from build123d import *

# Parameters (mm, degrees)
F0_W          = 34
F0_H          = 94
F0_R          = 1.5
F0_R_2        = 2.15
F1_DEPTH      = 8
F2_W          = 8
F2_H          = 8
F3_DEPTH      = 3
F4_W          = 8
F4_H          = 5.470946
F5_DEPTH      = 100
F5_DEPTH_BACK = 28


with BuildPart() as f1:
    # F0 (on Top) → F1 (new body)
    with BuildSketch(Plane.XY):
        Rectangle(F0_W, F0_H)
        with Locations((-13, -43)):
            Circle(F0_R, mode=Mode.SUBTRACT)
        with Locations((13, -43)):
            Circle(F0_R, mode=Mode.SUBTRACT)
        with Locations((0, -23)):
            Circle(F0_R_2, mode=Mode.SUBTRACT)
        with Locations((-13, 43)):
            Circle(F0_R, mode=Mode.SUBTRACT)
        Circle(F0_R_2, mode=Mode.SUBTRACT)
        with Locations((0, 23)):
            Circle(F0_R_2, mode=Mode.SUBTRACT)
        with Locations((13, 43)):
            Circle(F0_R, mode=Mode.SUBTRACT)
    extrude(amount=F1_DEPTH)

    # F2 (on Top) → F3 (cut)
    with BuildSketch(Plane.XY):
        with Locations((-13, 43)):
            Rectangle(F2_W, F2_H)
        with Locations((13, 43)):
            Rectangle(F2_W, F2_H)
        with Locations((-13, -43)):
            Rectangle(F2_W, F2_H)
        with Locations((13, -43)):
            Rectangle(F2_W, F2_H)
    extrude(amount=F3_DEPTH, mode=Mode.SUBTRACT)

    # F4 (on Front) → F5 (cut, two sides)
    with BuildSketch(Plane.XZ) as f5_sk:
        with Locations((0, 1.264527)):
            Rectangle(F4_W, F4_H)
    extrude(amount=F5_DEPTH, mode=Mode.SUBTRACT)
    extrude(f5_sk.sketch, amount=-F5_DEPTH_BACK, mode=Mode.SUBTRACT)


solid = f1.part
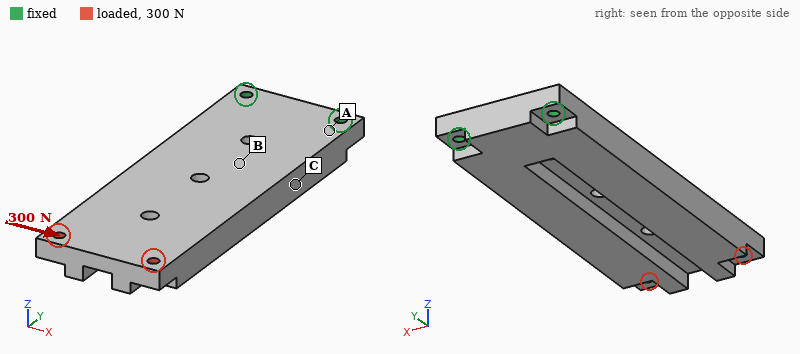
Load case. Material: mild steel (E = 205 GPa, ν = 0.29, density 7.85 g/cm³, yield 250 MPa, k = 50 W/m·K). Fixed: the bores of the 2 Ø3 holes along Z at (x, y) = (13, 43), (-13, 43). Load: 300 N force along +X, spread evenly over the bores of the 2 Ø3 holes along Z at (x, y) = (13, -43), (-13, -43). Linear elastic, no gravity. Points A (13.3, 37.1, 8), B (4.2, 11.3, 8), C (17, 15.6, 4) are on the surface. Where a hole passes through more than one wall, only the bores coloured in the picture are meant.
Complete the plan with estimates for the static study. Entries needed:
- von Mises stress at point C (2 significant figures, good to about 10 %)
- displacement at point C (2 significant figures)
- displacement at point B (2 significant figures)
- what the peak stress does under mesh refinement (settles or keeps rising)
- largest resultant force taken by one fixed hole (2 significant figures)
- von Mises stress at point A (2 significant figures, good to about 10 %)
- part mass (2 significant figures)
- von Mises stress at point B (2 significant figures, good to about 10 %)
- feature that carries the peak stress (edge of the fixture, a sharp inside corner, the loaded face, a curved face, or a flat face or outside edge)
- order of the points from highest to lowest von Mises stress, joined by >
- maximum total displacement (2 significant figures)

12 MPa
4.1 µm
4.0 µm
keeps rising
980 N
19 MPa
170 g
5.5 MPa
edge of the fixture
A > C > B
18 µm
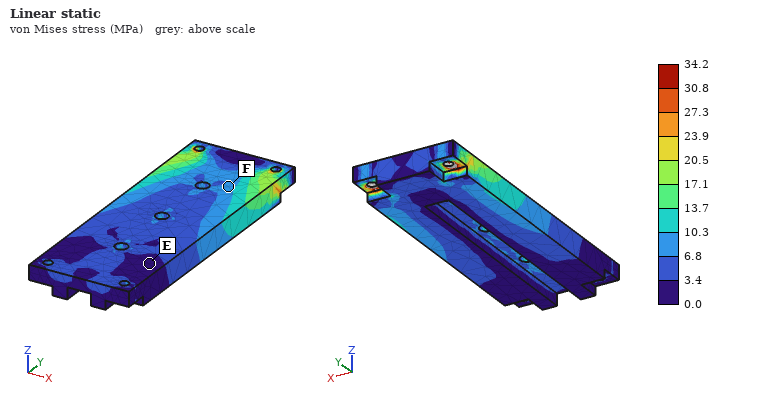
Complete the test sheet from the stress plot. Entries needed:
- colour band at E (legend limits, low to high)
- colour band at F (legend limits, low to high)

0.0 to 3.4 MPa
6.8 to 10.3 MPa
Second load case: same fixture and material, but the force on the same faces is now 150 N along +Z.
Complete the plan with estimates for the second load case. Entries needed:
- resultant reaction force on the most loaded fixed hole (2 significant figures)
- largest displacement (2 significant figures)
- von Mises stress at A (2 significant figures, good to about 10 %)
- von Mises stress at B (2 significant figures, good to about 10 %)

99 N
0.21 mm
61 MPa
23 MPa
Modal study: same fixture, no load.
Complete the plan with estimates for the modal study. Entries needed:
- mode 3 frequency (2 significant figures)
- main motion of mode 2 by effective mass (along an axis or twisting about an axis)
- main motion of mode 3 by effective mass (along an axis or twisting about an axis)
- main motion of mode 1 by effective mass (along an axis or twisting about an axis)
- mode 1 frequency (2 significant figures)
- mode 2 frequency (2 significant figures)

3400 Hz
along X
twisting about Y
along Z
640 Hz
3000 Hz
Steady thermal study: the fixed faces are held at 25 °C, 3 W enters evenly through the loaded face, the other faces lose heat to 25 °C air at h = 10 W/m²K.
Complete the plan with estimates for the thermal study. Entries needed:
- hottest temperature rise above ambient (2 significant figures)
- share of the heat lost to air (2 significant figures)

21 K
28 %
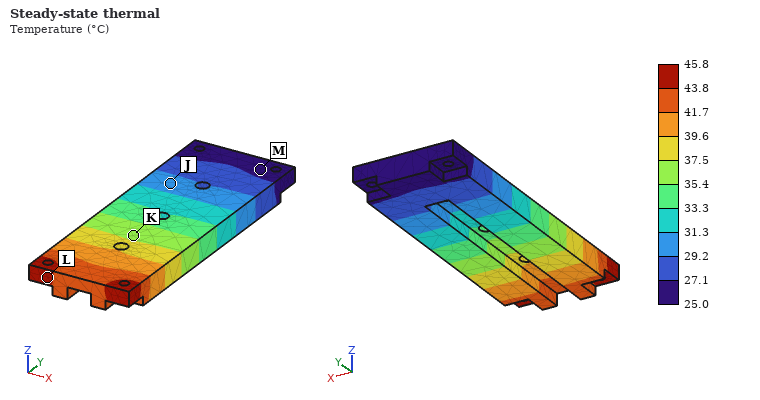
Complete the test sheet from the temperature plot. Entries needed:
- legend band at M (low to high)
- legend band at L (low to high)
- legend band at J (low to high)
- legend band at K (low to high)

25.0 to 27.1 °C
43.8 to 45.8 °C
29.2 to 31.3 °C
35.4 to 37.5 °C
